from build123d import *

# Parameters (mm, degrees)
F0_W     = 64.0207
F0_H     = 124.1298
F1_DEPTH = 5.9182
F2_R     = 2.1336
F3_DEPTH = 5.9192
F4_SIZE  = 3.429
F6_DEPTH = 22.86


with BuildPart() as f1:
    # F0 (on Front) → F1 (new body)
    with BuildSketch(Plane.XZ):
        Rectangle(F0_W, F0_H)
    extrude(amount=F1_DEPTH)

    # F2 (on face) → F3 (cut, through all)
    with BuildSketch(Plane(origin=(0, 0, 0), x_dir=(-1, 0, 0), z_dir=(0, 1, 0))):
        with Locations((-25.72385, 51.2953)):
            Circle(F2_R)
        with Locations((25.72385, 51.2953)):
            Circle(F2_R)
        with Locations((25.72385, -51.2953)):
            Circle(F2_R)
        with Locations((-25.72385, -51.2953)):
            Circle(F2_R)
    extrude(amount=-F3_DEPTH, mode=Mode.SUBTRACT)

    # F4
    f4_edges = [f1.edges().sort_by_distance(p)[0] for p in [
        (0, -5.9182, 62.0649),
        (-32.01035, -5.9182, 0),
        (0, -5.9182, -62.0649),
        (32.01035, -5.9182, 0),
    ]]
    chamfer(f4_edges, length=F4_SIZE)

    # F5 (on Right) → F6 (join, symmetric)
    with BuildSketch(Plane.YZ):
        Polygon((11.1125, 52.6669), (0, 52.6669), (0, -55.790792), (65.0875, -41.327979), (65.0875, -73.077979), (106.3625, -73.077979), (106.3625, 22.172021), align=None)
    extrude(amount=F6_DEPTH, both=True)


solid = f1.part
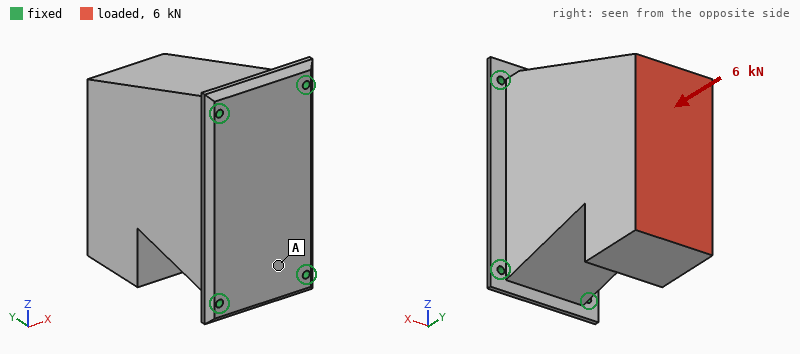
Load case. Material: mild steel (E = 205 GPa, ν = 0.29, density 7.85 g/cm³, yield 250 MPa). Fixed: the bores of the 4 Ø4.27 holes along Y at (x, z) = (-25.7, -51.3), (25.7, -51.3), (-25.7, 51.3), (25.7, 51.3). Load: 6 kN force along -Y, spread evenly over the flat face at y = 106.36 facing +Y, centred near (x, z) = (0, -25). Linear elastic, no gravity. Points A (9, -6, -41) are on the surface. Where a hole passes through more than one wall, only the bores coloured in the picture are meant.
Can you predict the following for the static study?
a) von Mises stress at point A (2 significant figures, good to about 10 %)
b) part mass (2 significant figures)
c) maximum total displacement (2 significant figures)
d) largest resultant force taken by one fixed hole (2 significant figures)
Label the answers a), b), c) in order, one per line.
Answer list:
a) 5.7 MPa
b) 4.1 kg
c) 8.6 µm
d) 2.5 kN
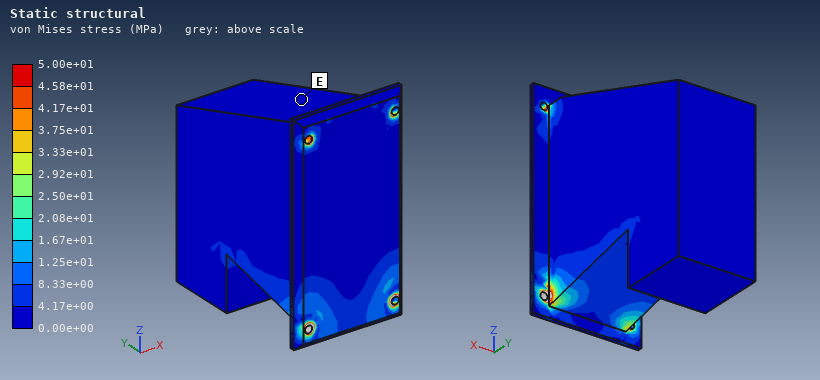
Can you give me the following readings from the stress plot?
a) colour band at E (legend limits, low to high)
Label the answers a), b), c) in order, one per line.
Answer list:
a) 0.00e+00 to 4.17e+00 MPa
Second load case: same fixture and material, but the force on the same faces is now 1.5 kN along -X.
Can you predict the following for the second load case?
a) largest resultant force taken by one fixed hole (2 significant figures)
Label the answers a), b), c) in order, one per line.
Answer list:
a) 2.0 kN
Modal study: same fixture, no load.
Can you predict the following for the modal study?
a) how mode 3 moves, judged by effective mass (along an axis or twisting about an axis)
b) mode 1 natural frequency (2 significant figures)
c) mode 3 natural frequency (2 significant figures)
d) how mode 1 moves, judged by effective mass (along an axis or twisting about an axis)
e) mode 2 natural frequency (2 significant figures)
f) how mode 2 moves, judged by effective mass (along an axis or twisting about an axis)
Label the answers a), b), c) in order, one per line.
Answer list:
a) along Y
b) 1200 Hz
c) 3500 Hz
d) along X
e) 2400 Hz
f) along Z
